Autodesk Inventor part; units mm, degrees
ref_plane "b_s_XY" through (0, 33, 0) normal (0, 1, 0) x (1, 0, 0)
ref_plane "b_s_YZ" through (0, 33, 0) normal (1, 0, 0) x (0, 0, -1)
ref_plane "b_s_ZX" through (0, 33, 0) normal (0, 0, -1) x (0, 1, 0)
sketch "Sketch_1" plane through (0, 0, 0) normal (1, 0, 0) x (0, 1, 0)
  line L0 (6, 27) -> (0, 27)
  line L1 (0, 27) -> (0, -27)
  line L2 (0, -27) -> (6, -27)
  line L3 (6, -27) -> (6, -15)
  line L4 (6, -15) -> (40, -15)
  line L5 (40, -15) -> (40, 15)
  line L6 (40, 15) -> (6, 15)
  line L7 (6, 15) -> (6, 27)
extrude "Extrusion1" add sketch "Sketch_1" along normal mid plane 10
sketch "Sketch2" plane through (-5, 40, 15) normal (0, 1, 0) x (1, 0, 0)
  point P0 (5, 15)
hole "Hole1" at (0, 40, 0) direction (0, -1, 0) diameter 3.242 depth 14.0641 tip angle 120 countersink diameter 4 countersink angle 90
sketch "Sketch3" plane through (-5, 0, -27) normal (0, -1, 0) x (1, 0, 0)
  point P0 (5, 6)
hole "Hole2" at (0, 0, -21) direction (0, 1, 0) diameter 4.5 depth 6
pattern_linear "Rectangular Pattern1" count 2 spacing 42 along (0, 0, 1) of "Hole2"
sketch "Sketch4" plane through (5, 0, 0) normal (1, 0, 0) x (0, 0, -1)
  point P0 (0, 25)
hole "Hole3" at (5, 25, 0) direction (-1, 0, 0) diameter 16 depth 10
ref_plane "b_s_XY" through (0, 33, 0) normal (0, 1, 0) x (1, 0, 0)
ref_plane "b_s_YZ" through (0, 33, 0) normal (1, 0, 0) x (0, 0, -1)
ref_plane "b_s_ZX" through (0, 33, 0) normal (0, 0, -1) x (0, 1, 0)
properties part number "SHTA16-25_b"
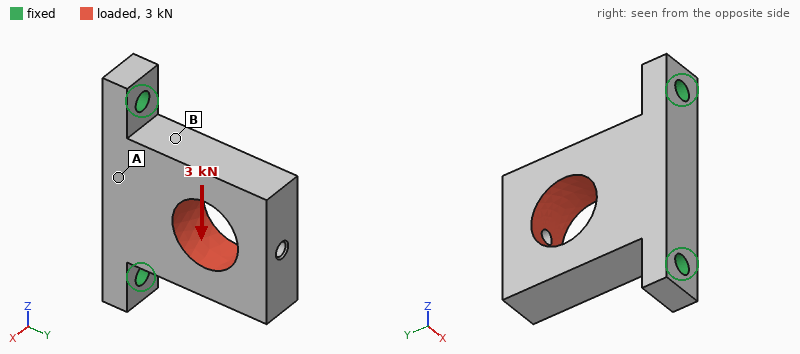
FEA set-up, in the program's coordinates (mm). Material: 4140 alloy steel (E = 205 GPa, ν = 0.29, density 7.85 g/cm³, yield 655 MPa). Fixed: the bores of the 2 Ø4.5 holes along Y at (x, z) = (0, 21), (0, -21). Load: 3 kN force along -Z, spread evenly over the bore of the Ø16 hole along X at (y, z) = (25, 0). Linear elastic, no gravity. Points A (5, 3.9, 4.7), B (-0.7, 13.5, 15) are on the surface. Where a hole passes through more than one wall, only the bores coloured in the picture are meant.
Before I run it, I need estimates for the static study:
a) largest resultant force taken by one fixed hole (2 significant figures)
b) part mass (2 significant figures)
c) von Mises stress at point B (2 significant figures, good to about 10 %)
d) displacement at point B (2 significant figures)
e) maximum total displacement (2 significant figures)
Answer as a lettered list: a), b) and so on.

a) 2.4 kN
b) 88 g
c) 43 MPa
d) 7.8 µm
e) 24 µm
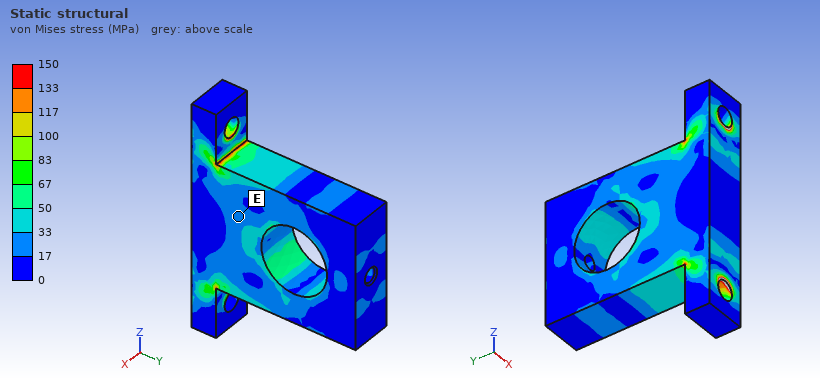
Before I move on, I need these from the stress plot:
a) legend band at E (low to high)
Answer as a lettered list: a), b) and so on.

a) 17 to 33 MPa
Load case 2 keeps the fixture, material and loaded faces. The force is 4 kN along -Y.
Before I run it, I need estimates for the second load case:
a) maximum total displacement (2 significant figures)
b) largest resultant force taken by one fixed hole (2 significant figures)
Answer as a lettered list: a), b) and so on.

a) 9.1 µm
b) 2.2 kN
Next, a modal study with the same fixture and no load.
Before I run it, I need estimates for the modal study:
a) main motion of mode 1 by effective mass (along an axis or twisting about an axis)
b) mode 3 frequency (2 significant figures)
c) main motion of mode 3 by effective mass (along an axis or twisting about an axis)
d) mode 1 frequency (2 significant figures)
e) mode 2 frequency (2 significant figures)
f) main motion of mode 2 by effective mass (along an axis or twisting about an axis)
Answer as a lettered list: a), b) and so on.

a) along X
b) 10 kHz
c) twisting about Y
d) 2700 Hz
e) 8500 Hz
f) along Z
